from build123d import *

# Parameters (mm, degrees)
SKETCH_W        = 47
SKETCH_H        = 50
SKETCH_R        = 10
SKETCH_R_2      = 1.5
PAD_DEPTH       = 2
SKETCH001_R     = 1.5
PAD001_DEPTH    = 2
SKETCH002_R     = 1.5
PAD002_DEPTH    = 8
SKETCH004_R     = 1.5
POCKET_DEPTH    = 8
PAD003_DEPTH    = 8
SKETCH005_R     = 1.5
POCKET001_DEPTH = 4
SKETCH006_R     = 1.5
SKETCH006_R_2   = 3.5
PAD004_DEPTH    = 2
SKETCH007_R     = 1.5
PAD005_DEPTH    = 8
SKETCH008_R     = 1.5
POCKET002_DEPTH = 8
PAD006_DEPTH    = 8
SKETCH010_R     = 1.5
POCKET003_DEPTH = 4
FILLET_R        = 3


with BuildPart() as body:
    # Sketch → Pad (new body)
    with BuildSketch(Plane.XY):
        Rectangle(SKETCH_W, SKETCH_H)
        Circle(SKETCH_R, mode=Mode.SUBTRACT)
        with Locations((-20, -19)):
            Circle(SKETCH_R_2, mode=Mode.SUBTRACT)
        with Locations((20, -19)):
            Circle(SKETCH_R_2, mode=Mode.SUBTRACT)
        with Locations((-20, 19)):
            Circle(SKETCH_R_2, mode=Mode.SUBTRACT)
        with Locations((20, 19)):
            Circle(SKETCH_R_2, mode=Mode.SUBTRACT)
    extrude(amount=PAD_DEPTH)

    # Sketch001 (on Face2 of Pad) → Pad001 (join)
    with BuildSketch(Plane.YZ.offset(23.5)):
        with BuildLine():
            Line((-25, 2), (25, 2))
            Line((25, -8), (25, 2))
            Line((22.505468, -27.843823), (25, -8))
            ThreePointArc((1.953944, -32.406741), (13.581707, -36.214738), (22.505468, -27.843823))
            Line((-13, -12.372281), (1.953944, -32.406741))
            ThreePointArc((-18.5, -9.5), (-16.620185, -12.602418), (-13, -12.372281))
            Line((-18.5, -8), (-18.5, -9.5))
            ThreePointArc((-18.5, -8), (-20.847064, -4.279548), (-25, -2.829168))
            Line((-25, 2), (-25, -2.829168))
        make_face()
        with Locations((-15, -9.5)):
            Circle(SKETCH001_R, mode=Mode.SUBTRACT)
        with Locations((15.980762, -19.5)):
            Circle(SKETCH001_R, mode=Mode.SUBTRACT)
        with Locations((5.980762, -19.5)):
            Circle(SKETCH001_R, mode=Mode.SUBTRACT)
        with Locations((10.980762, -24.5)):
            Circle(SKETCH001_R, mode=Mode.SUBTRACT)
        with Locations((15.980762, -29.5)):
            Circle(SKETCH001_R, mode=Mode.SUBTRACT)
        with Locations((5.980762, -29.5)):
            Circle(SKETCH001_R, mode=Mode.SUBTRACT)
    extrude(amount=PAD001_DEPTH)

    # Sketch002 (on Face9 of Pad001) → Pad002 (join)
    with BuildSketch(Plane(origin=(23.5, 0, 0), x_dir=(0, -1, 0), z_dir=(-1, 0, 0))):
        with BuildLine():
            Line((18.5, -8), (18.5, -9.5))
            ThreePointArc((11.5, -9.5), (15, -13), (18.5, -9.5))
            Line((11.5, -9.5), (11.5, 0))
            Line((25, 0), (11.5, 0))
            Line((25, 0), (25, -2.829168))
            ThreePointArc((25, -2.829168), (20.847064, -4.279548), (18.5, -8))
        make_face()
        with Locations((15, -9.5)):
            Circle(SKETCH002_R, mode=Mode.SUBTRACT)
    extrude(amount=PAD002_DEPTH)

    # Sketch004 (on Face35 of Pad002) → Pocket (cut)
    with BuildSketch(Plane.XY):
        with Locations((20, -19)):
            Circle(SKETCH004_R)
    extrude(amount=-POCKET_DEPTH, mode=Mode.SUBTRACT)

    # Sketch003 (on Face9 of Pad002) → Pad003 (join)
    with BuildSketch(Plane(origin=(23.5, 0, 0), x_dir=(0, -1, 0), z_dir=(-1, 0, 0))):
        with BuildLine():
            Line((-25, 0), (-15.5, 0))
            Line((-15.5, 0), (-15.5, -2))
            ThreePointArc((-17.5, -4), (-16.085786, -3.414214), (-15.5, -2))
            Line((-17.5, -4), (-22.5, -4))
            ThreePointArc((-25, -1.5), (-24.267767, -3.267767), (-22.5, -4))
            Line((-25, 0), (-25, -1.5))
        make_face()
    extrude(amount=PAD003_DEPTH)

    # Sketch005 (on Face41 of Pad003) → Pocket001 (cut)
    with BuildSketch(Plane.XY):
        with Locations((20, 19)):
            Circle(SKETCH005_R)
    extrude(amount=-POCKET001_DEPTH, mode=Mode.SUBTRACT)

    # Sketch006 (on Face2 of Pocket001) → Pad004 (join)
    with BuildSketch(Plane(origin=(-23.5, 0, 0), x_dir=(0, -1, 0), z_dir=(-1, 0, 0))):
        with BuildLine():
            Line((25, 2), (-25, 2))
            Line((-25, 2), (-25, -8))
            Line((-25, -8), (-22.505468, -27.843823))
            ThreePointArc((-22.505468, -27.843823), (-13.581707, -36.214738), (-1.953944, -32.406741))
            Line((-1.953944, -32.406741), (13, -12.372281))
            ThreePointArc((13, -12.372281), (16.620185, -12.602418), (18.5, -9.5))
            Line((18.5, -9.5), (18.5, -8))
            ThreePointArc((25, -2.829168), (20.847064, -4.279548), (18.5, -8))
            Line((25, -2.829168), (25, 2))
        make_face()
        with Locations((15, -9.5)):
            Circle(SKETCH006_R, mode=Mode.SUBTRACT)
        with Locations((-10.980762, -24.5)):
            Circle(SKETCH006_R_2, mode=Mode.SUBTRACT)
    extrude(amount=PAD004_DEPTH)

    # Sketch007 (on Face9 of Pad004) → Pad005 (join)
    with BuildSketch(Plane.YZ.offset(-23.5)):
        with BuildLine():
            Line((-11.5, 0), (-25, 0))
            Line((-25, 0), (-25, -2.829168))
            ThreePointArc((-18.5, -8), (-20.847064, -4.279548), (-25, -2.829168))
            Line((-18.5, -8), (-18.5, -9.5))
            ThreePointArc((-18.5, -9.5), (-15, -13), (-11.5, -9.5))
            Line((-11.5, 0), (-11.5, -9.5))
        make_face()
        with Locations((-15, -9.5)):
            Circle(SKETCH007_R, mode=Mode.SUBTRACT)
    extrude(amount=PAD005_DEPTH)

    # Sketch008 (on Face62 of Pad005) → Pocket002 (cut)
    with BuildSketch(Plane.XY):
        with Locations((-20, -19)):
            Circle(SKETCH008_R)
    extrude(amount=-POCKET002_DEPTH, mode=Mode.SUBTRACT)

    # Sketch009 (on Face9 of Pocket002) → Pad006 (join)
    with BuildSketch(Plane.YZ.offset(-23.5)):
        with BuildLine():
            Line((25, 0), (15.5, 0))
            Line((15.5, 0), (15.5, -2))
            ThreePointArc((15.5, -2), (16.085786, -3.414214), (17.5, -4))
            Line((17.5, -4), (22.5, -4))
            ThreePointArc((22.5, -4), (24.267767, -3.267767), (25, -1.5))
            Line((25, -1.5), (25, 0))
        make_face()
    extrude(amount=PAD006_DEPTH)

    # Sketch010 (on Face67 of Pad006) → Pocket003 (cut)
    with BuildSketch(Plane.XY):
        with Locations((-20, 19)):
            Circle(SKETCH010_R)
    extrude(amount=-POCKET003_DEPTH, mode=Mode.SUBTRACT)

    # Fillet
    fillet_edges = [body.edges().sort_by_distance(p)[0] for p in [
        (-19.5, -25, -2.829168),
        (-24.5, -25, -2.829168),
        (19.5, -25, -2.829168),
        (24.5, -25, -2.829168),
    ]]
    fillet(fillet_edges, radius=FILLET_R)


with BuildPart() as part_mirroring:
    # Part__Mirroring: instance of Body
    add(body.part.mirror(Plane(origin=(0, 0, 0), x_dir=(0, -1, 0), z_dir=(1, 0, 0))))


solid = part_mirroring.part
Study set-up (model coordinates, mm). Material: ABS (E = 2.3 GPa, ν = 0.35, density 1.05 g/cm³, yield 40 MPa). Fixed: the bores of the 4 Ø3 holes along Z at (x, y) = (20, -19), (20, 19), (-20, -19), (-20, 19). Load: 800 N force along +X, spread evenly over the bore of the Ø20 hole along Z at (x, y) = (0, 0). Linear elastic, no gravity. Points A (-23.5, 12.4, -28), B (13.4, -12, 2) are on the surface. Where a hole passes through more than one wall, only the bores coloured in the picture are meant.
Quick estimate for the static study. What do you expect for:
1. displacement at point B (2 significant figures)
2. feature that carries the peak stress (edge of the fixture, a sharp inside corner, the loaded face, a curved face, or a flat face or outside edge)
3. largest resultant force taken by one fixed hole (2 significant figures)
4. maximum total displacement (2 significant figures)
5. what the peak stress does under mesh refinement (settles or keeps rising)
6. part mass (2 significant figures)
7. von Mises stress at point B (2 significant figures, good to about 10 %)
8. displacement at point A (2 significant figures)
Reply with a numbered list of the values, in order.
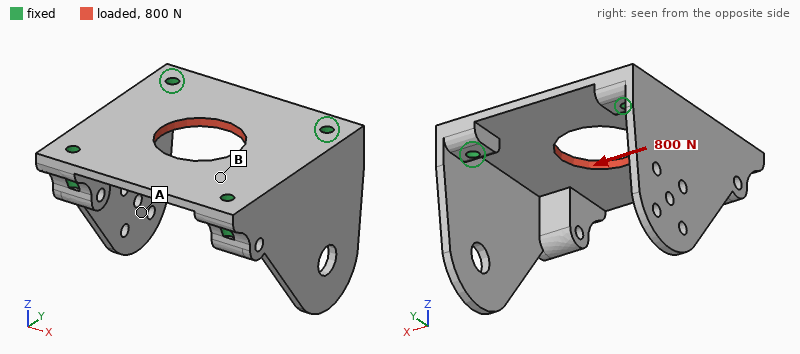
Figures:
1. 0.045 mm
2. edge of the fixture
3. 210 N
4. 0.10 mm
5. keeps rising
6. 12 g
7. 6.7 MPa
8. 0.042 mm
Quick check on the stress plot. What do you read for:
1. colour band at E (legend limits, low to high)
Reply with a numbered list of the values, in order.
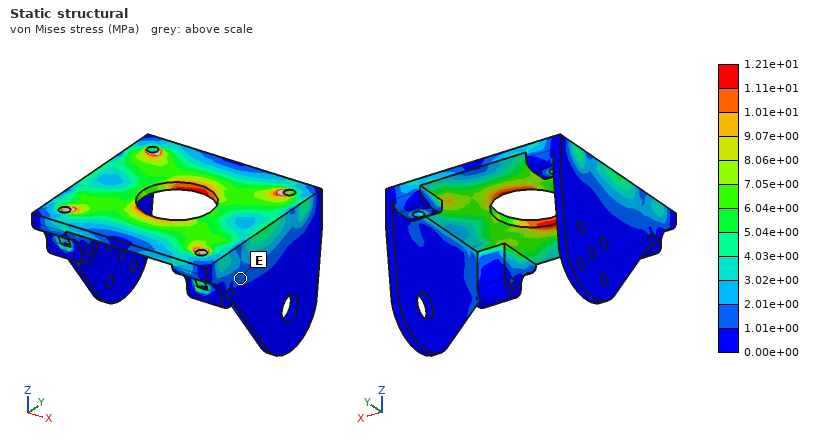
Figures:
1. 1.01e+00 to 2.01e+00 MPa
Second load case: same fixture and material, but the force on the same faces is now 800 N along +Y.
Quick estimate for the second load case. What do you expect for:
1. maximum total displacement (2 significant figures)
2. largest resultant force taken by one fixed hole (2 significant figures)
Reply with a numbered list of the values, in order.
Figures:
1. 0.11 mm
2. 230 N
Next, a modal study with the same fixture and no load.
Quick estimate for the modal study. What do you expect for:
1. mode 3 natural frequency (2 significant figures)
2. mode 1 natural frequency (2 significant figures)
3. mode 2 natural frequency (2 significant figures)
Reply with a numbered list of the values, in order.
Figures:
1. 1800 Hz
2. 580 Hz
3. 580 Hz
